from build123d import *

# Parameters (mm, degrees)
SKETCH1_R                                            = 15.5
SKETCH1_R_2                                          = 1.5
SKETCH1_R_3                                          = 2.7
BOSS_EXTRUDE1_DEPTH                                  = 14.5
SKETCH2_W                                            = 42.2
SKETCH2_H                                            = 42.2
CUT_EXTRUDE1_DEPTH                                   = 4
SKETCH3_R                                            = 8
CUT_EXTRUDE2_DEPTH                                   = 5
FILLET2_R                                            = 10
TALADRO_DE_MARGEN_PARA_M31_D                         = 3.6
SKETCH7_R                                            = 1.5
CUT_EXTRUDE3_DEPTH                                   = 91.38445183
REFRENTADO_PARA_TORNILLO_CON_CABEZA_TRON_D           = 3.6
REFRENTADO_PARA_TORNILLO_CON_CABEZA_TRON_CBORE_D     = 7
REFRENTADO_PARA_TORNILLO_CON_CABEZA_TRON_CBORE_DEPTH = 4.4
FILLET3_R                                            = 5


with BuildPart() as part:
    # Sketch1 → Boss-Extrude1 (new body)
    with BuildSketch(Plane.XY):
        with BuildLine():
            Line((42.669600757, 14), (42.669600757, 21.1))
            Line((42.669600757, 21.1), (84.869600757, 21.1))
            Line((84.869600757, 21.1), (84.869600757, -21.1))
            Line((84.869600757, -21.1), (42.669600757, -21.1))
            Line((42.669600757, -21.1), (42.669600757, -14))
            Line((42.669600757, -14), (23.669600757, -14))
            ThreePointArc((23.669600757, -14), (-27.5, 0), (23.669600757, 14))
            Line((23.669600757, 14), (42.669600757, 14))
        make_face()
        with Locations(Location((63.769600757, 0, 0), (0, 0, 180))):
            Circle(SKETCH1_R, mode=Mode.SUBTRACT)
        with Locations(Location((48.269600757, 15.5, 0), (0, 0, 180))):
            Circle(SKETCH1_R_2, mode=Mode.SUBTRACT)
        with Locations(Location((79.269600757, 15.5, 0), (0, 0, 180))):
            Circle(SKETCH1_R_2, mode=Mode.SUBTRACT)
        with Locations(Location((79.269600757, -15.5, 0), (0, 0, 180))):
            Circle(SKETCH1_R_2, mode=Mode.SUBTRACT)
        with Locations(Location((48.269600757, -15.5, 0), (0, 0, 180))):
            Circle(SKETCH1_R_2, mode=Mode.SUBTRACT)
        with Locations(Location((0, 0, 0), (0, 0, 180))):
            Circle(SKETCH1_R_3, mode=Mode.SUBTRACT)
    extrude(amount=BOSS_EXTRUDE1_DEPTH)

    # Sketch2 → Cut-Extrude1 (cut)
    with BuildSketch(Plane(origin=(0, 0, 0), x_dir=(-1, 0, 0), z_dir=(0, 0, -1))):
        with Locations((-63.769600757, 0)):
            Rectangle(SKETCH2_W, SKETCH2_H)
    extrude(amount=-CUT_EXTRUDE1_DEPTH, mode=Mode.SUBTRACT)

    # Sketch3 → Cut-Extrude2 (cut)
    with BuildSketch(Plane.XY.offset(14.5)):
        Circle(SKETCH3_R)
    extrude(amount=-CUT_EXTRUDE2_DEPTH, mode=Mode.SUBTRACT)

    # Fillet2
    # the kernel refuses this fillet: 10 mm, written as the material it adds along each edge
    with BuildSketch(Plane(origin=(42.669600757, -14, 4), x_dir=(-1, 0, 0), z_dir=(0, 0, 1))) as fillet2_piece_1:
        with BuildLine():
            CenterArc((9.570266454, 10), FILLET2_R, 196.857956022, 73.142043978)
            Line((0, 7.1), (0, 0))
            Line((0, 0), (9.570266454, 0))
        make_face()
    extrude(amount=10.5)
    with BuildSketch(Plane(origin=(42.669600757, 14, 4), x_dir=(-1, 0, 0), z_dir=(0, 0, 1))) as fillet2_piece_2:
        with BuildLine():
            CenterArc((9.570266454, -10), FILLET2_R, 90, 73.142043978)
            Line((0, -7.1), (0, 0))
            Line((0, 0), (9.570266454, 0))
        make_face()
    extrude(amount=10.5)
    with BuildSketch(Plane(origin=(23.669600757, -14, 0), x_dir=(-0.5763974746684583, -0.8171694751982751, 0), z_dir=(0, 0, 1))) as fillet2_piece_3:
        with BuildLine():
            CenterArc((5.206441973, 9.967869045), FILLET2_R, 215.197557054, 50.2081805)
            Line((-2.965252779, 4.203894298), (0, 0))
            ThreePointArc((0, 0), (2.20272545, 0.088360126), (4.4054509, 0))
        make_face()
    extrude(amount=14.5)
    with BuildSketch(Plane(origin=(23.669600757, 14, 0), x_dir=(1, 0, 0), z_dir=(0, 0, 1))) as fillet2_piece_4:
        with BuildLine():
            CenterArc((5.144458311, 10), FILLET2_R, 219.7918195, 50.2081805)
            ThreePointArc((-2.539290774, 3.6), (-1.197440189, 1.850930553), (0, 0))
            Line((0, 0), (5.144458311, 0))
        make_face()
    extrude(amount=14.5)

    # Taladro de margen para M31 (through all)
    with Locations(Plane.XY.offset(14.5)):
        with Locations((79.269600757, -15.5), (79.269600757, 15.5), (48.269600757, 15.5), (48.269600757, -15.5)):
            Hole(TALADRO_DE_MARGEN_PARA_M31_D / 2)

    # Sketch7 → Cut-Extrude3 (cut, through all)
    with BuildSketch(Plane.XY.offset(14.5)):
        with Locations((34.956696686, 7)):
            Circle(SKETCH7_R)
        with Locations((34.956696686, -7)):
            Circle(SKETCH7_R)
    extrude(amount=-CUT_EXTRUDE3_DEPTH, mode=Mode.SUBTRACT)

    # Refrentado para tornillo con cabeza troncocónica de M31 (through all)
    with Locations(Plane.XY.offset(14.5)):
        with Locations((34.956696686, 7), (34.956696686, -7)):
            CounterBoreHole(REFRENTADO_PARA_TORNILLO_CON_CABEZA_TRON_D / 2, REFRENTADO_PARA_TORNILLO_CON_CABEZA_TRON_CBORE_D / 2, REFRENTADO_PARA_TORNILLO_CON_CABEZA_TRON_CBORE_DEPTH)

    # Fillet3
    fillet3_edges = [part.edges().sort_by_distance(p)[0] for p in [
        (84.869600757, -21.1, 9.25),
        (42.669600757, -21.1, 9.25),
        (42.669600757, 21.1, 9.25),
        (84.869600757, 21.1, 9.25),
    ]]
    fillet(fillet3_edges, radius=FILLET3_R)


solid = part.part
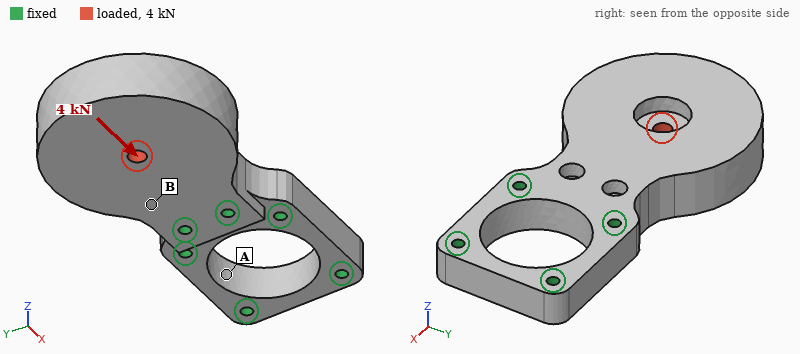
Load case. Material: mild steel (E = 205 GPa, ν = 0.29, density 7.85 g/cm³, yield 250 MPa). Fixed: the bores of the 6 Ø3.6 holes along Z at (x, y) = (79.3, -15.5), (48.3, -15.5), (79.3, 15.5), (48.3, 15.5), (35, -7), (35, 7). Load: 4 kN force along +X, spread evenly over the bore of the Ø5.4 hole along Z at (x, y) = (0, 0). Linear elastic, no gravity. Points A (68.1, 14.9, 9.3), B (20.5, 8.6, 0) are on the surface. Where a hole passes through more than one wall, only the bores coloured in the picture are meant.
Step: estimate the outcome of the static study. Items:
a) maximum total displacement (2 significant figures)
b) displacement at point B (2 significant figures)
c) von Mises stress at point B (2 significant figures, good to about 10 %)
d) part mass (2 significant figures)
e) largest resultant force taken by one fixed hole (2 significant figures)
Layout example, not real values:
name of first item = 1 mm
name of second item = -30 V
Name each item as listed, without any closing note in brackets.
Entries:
maximum total displacement = 8.6 µm
displacement at point B = 1.6 µm
von Mises stress at point B = 18 MPa
part mass = 390 g
largest resultant force taken by one fixed hole = 1.8 kN
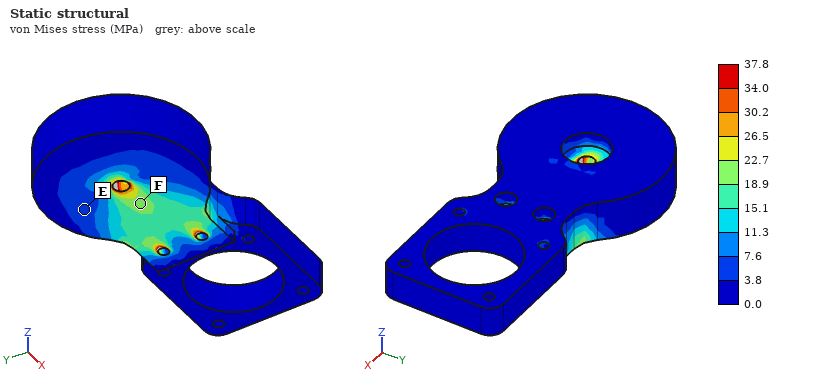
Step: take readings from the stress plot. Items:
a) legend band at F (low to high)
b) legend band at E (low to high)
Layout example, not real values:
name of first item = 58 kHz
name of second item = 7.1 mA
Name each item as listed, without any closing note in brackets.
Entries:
legend band at F = 18.9 to 22.7 MPa
legend band at E = 3.8 to 7.6 MPa
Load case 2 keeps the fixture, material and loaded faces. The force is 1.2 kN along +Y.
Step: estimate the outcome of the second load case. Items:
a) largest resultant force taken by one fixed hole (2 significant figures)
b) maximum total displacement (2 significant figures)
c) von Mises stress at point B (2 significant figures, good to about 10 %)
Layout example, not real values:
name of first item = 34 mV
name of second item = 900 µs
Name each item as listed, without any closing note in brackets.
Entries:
largest resultant force taken by one fixed hole = 1.8 kN
maximum total displacement = 9.7 µm
von Mises stress at point B = 12 MPa
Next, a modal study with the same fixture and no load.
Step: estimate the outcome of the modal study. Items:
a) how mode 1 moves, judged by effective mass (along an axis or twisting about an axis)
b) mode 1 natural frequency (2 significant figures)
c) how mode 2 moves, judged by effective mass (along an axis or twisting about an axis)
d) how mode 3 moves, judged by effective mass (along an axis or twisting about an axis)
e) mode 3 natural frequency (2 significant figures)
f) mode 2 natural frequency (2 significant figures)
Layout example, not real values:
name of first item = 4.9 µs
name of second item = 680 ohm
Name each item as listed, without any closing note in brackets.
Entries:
how mode 1 moves, judged by effective mass = along Z
mode 1 natural frequency = 2300 Hz
how mode 2 moves, judged by effective mass = along Y
how mode 3 moves, judged by effective mass = twisting about X
mode 3 natural frequency = 5500 Hz
mode 2 natural frequency = 4100 Hz
